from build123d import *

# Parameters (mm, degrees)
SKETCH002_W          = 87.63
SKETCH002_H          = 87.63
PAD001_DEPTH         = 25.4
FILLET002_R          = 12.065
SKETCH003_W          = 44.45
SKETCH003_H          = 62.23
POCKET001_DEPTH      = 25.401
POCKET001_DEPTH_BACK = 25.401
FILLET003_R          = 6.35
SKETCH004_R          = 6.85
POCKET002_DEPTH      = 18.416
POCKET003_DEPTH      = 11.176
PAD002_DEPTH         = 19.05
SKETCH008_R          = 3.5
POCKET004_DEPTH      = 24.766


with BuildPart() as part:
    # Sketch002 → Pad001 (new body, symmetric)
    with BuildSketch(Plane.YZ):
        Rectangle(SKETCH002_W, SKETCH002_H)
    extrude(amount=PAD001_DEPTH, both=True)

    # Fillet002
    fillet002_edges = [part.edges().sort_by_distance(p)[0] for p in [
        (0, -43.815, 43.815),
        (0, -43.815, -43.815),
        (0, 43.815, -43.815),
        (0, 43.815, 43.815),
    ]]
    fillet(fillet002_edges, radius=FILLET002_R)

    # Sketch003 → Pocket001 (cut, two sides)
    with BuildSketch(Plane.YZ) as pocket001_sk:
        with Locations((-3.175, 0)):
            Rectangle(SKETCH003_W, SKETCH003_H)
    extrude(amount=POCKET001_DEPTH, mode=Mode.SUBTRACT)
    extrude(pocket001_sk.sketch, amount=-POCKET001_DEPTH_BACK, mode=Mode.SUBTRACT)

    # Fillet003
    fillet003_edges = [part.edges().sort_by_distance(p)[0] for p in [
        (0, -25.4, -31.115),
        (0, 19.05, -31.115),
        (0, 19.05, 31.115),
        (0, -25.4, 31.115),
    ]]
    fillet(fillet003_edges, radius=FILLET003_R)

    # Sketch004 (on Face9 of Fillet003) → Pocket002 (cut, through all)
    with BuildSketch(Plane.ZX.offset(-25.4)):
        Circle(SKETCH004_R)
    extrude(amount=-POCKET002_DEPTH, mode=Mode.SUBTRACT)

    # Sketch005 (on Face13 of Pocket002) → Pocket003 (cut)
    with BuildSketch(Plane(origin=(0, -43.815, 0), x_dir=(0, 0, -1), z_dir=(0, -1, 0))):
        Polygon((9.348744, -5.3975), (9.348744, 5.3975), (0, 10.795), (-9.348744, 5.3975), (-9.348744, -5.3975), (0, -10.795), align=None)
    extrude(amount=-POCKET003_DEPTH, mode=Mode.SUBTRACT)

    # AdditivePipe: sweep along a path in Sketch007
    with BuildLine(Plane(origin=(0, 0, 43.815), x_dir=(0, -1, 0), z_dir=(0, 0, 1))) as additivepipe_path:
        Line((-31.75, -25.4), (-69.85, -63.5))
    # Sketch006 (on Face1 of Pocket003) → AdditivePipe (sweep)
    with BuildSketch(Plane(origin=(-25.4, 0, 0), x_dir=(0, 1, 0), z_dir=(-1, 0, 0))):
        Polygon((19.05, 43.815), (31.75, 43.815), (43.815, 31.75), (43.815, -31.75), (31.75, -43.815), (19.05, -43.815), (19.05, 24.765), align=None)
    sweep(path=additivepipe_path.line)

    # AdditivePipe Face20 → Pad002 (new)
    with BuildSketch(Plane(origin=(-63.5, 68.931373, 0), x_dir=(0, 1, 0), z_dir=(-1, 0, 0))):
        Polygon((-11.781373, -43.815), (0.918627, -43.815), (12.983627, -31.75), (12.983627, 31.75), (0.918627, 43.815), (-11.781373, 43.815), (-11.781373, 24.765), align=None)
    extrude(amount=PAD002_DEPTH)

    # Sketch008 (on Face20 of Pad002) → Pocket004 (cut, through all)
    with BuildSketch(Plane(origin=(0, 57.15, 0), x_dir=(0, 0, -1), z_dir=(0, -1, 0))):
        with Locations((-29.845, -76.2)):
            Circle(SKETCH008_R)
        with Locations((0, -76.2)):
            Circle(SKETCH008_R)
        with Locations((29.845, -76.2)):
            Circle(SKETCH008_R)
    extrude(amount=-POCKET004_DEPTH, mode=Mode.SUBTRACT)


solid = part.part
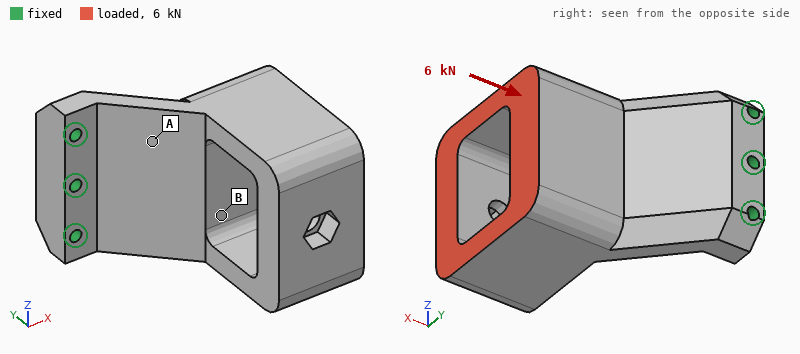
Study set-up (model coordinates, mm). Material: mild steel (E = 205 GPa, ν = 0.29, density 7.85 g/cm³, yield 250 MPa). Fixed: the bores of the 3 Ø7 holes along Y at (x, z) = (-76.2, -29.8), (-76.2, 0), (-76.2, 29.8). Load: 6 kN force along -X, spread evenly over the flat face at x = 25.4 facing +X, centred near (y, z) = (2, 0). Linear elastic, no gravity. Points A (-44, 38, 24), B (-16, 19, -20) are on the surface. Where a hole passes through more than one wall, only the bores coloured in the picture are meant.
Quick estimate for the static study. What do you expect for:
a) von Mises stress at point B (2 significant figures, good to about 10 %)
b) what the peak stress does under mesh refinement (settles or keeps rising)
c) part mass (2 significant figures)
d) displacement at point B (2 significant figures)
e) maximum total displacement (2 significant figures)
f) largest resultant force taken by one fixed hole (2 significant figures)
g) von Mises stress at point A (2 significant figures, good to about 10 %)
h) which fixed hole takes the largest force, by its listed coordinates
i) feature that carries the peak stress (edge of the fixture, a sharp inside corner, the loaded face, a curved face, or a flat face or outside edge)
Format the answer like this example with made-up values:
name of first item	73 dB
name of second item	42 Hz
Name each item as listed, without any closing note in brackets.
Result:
von Mises stress at point B	15 MPa
what the peak stress does under mesh refinement	keeps rising
part mass	2.8 kg
displacement at point B	0.11 mm
maximum total displacement	0.30 mm
largest resultant force taken by one fixed hole	2.8 kN
von Mises stress at point A	59 MPa
which fixed hole takes the largest force, by its listed coordinates	(-76.2, 0)
feature that carries the peak stress	edge of the fixture
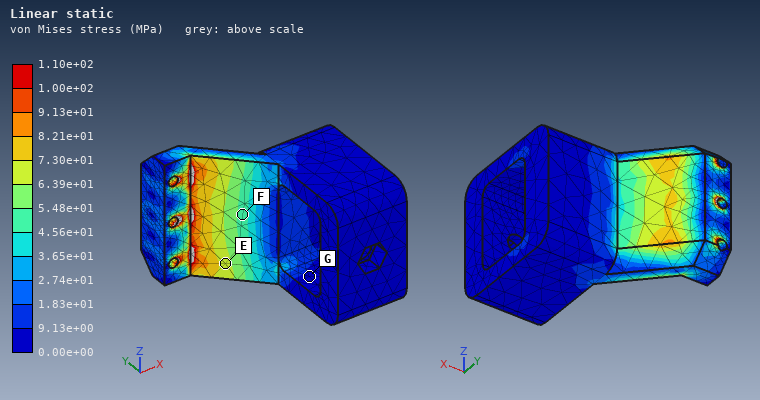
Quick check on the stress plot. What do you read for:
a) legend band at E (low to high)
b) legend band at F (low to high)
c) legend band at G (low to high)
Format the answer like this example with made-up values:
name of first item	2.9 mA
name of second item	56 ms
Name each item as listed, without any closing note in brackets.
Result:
legend band at E	6.39e+01 to 7.30e+01 MPa
legend band at F	4.56e+01 to 5.48e+01 MPa
legend band at G	0.00e+00 to 9.13e+00 MPa
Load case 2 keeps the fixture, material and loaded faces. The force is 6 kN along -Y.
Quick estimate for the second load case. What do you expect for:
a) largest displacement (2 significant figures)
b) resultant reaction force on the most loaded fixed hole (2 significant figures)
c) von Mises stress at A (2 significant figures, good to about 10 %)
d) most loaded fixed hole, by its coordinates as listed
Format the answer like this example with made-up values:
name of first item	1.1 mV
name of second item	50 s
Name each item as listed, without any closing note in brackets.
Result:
largest displacement	0.43 mm
resultant reaction force on the most loaded fixed hole	4.1 kN
von Mises stress at A	81 MPa
most loaded fixed hole, by its coordinates as listed	(-76.2, 0)
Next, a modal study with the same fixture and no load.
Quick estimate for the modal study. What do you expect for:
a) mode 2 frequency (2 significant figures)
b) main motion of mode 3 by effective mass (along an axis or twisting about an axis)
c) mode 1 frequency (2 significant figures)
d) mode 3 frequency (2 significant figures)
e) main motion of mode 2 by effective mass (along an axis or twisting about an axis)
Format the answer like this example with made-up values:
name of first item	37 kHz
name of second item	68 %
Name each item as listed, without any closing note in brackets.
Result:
mode 2 frequency	1300 Hz
main motion of mode 3 by effective mass	along Z
mode 1 frequency	530 Hz
mode 3 frequency	2100 Hz
main motion of mode 2 by effective mass	along Z
